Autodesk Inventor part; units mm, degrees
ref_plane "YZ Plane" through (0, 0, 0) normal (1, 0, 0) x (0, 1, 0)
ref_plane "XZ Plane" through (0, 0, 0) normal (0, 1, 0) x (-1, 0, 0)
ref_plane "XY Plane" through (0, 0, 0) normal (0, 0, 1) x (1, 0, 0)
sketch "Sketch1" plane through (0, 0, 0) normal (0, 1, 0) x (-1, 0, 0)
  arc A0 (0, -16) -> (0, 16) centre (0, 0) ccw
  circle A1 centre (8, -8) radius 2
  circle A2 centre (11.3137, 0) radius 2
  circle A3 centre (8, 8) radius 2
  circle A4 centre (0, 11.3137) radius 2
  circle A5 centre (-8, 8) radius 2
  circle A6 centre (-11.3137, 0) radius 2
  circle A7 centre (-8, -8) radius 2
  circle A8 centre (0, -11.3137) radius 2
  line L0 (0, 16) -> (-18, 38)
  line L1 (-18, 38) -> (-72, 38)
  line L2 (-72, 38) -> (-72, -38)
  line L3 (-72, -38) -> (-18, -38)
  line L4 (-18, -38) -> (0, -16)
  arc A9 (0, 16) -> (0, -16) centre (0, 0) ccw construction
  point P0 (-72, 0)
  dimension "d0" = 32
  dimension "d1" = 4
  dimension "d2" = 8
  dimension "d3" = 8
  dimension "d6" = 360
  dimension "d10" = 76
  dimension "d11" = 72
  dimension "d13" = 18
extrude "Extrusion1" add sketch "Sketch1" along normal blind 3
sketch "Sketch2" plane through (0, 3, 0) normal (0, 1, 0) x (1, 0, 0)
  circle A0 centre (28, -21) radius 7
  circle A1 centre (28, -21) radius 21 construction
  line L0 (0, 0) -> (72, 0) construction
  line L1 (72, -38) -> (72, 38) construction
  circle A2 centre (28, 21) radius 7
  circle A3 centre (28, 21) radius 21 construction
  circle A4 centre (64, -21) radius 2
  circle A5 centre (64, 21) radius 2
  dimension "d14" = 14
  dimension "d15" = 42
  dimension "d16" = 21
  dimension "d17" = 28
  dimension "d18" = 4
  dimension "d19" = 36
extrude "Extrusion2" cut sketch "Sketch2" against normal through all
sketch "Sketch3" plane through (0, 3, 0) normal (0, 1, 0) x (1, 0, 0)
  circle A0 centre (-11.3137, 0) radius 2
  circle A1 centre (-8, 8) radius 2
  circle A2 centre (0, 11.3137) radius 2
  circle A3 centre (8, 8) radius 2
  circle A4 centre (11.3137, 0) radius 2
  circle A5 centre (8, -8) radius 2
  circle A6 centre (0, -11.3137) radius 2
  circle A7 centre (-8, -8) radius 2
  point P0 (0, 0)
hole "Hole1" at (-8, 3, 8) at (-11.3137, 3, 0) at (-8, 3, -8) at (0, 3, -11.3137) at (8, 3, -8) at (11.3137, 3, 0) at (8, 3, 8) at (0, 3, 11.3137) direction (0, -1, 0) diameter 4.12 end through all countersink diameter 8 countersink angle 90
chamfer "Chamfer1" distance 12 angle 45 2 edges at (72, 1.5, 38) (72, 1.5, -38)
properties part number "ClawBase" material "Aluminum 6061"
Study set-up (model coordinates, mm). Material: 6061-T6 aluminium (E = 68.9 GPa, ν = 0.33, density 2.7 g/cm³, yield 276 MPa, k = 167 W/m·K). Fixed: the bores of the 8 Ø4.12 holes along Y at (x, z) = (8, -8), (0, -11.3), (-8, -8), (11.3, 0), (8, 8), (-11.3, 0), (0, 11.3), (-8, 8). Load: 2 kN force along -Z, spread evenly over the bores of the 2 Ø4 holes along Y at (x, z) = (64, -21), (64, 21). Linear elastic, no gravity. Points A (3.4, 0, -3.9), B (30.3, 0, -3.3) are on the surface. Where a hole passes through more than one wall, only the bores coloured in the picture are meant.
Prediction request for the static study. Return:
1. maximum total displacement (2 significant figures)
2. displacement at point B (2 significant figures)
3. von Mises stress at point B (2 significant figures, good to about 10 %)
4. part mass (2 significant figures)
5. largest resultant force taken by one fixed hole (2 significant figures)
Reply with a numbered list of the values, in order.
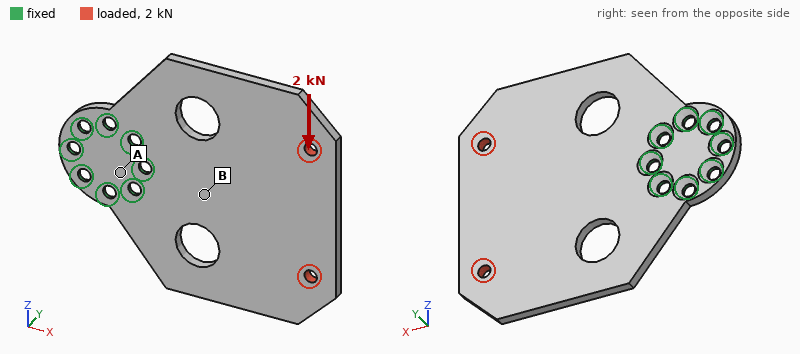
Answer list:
1. 0.21 mm
2. 0.061 mm
3. 56 MPa
4. 39 g
5. 2.3 kN
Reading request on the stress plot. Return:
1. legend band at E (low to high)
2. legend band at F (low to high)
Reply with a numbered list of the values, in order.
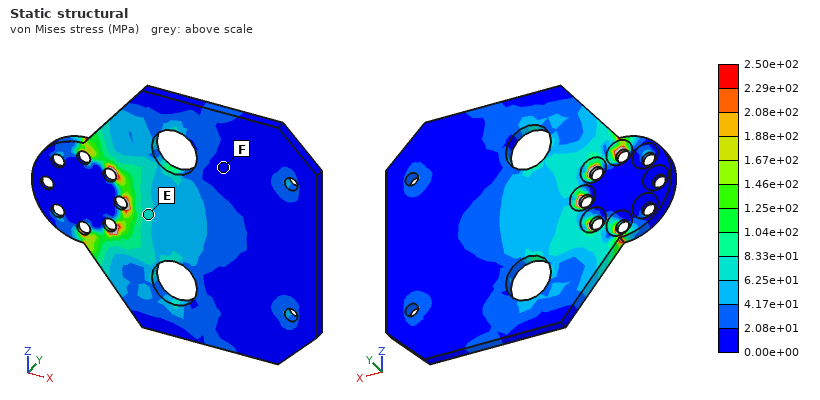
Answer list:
1. 6.25e+01 to 8.33e+01 MPa
2. 0.00e+00 to 2.08e+01 MPa
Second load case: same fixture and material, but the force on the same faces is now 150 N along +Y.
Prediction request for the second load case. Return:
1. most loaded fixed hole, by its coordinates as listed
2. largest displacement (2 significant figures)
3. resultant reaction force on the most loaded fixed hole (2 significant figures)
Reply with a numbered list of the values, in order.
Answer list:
1. (11.3, 0)
2. 1.3 mm
3. 700 N
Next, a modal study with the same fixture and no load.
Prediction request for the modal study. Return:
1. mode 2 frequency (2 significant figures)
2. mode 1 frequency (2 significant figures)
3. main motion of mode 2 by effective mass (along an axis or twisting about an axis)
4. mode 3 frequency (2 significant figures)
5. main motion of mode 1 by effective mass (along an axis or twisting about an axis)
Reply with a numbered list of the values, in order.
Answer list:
1. 930 Hz
2. 510 Hz
3. twisting about X
4. 2300 Hz
5. along Y
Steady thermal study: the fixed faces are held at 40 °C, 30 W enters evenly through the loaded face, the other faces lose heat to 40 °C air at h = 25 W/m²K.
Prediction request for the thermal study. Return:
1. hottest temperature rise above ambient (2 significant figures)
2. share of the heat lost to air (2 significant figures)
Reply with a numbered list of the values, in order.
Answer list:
1. 57 K
2. 25 %
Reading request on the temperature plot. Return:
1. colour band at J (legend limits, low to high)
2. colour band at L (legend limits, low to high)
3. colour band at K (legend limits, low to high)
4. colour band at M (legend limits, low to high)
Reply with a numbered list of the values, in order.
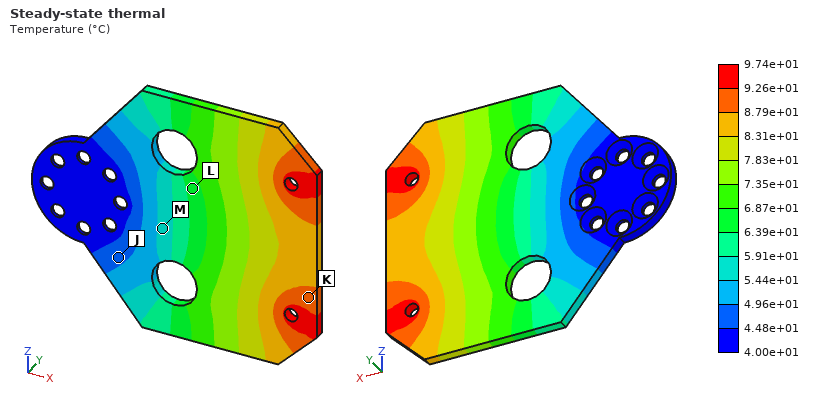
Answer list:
1. 4.48e+01 to 4.96e+01 °C
2. 6.39e+01 to 6.87e+01 °C
3. 8.79e+01 to 9.26e+01 °C
4. 5.44e+01 to 5.91e+01 °C
